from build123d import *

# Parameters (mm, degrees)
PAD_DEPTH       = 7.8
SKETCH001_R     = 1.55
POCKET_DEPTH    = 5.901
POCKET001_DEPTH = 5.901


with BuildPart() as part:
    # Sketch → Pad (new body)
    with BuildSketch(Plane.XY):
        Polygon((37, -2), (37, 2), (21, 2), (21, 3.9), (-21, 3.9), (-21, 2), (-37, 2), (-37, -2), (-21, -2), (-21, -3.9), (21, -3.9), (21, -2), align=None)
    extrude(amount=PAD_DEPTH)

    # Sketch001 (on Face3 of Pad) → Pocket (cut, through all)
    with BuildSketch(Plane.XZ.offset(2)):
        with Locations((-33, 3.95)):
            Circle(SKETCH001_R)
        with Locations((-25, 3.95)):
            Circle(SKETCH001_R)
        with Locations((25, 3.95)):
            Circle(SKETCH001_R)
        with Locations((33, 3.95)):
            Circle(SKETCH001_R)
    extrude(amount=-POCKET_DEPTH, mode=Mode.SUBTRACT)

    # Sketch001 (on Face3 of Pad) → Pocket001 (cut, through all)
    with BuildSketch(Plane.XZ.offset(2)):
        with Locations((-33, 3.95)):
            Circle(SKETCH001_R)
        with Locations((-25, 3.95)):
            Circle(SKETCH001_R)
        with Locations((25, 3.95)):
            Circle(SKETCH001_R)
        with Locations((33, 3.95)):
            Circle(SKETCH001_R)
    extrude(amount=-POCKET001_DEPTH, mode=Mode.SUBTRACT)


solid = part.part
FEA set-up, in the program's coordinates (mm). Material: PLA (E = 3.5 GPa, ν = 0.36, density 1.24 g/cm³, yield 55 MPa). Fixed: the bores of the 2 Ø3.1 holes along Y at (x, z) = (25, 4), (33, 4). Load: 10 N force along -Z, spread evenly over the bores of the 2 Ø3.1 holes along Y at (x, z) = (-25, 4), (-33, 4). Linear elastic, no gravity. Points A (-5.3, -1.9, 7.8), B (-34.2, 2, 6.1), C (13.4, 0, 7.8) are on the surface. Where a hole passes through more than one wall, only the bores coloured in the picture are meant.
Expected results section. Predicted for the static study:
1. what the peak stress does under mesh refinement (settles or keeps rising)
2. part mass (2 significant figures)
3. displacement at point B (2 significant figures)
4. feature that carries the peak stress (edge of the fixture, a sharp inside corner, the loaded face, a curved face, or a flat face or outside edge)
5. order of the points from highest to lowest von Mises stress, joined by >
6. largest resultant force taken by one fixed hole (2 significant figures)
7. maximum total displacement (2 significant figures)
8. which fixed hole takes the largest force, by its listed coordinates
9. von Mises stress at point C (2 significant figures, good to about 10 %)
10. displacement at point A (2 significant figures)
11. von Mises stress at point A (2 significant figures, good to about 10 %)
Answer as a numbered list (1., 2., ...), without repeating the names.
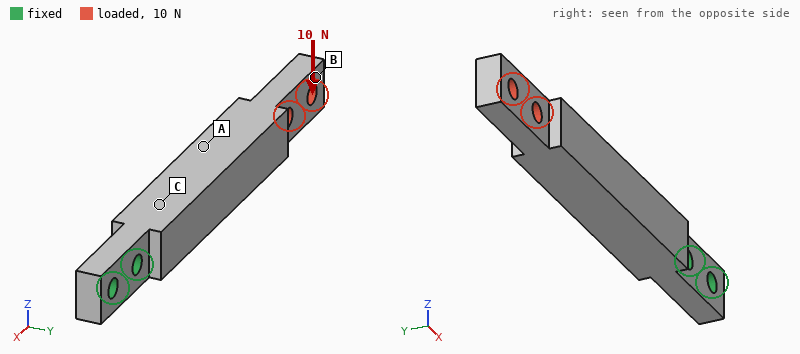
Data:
1. keeps rising
2. 4.3 g
3. 0.80 mm
4. edge of the fixture
5. C > A > B
6. 33 N
7. 0.85 mm
8. (25, 4)
9. 5.5 MPa
10. 0.31 mm
11. 3.0 MPa
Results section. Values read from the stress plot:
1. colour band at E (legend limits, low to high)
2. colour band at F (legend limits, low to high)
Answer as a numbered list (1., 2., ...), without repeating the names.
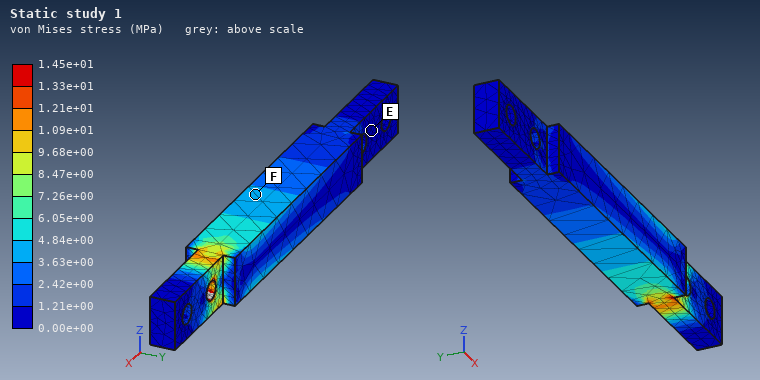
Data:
1. 0.00e+00 to 1.21e+00 MPa
2. 3.63e+00 to 4.84e+00 MPa
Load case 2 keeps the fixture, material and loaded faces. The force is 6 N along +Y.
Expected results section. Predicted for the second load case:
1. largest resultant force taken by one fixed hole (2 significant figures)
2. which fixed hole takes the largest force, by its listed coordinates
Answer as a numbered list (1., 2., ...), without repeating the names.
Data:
1. 11 N
2. (25, 4)
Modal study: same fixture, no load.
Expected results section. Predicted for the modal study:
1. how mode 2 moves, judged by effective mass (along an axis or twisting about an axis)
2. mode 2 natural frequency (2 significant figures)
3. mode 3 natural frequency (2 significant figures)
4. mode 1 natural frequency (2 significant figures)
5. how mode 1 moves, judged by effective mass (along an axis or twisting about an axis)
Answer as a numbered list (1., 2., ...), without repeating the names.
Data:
1. along Z
2. 560 Hz
3. 2700 Hz
4. 430 Hz
5. along Y
